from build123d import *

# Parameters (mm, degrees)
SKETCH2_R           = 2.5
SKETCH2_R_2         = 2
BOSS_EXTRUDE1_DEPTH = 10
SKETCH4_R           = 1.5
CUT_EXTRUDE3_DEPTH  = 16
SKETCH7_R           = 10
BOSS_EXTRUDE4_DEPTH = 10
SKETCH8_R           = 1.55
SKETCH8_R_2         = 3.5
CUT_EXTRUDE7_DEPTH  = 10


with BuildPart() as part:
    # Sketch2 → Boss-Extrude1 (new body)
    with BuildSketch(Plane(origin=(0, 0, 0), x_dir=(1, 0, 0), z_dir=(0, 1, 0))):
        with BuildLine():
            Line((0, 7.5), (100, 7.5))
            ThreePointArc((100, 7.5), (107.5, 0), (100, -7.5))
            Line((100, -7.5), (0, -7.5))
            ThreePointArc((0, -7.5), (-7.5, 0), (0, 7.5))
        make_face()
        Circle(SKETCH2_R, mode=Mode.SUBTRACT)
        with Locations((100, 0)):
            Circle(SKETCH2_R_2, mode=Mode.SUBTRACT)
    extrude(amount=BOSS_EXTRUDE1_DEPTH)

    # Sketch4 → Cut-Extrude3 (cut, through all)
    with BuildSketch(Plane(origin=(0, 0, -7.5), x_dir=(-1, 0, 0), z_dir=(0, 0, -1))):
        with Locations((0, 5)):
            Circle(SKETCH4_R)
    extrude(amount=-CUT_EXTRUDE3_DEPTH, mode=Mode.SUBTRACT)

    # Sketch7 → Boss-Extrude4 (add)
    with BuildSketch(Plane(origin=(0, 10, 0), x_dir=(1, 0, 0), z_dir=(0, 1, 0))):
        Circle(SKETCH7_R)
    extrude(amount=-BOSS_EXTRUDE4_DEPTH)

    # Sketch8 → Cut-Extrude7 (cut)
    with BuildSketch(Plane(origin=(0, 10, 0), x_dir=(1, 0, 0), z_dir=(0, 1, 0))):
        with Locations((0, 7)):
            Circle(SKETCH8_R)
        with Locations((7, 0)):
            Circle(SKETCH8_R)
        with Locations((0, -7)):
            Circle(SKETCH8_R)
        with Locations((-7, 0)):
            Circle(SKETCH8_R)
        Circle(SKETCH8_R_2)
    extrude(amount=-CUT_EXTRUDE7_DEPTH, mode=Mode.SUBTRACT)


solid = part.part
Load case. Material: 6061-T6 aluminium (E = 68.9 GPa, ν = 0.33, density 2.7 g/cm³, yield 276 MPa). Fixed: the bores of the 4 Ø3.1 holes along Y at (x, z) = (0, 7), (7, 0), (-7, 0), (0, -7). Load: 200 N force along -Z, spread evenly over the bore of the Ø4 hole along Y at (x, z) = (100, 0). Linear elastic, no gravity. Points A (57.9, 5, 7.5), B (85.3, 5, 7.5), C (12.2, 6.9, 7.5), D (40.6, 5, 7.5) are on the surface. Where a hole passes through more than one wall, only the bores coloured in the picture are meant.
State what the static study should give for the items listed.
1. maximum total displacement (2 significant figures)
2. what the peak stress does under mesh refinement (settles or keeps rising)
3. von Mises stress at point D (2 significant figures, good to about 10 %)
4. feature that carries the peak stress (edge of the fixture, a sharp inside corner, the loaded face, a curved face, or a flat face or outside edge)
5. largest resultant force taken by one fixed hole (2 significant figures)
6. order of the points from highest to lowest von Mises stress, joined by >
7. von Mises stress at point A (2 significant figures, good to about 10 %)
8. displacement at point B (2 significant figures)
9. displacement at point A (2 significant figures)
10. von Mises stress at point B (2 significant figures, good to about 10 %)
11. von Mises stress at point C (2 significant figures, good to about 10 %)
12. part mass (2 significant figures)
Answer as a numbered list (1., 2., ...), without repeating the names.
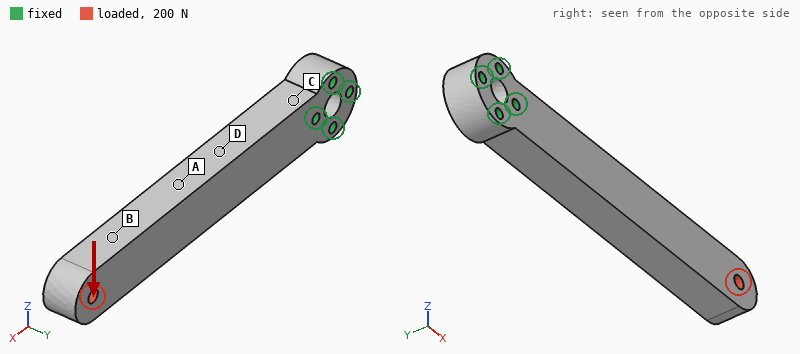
1. 0.35 mm
2. keeps rising
3. 32 MPa
4. a sharp inside corner
5. 1.1 kN
6. C > D > A > B
7. 22 MPa
8. 0.25 mm
9. 0.13 mm
10. 7.8 MPa
11. 47 MPa
12. 46 g
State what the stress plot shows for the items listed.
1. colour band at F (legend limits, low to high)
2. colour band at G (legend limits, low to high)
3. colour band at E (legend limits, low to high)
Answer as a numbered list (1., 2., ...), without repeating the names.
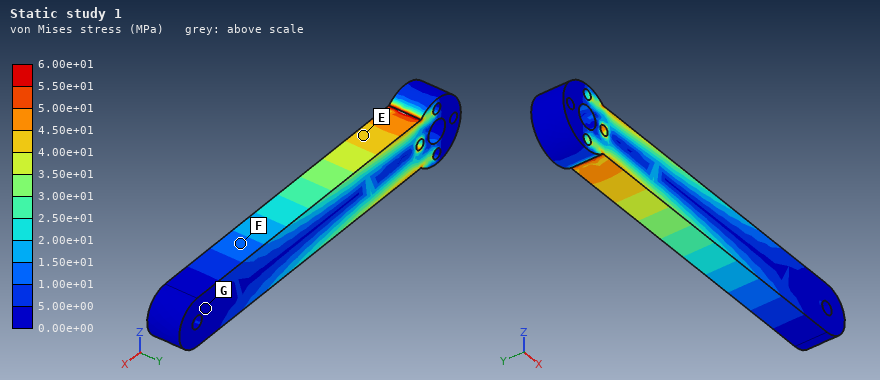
1. 1.00e+01 to 1.50e+01 MPa
2. 0.00e+00 to 5.00e+00 MPa
3. 4.00e+01 to 4.50e+01 MPa
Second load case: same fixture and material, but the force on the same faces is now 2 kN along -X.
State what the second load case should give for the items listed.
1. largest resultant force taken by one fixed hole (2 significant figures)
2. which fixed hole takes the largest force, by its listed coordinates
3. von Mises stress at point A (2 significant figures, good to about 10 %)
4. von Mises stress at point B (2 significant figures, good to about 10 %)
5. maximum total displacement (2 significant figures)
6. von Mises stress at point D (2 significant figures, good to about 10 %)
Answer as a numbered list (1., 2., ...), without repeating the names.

1. 1.3 kN
2. (7, 0)
3. 13 MPa
4. 13 MPa
5. 20 µm
6. 13 MPa
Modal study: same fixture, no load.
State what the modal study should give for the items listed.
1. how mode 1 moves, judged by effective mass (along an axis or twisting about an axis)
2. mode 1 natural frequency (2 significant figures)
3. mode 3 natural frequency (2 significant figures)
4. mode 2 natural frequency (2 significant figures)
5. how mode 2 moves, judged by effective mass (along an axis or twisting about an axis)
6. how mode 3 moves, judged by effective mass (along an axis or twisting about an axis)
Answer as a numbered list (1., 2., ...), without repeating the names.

1. along Y
2. 830 Hz
3. 4900 Hz
4. 1200 Hz
5. along Z
6. along Y
